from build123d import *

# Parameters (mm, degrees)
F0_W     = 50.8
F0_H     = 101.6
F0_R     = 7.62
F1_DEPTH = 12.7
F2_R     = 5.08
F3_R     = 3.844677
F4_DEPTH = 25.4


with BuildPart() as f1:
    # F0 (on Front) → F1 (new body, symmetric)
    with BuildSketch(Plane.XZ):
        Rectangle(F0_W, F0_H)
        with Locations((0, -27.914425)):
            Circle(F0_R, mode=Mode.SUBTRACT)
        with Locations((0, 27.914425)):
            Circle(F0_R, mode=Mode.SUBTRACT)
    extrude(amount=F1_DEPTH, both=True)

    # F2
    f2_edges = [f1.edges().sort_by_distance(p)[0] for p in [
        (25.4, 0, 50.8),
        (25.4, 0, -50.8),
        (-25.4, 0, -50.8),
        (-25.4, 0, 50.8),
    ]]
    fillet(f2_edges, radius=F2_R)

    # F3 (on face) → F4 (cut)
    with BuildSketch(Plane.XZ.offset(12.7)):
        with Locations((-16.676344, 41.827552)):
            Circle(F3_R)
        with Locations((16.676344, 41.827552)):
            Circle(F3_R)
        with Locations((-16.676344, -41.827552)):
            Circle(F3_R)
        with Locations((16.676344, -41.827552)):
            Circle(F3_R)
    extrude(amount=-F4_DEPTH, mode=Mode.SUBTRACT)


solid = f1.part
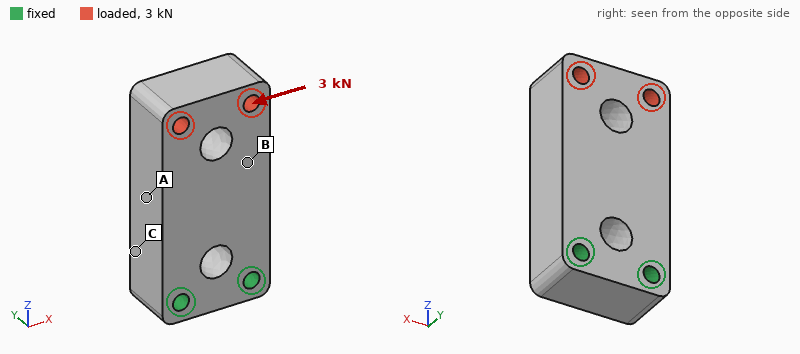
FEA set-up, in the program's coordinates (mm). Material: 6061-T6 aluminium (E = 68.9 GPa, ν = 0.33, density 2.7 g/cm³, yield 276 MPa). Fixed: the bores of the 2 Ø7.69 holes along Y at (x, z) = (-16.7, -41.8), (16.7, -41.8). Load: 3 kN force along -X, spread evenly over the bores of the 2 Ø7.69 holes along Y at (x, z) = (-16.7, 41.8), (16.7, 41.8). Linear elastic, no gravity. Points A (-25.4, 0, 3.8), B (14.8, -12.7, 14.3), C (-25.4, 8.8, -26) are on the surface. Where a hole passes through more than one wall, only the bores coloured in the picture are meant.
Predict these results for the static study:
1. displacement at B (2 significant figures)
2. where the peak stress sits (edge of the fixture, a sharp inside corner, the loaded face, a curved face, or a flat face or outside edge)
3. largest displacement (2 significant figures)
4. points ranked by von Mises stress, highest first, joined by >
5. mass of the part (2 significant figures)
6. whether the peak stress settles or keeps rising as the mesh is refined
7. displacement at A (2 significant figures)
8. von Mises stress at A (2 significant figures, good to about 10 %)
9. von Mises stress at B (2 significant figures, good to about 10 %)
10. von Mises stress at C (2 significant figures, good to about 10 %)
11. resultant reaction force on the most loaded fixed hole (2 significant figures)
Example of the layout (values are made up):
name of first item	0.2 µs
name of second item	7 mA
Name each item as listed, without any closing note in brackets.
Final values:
displacement at B	25 µm
where the peak stress sits	edge of the fixture
largest displacement	51 µm
points ranked by von Mises stress, highest first, joined by >	C > A > B
mass of the part	310 g
whether the peak stress settles or keeps rising as the mesh is refined	keeps rising
displacement at A	22 µm
von Mises stress at A	11 MPa
von Mises stress at B	4.9 MPa
von Mises stress at C	17 MPa
resultant reaction force on the most loaded fixed hole	6.6 kN
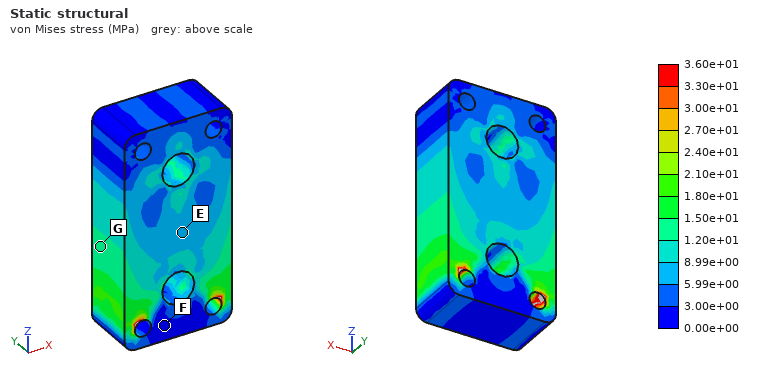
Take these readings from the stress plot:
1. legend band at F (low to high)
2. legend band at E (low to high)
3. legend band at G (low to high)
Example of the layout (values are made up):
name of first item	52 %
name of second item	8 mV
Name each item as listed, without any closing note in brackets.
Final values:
legend band at F	0.00e+00 to 3.00e+00 MPa
legend band at E	5.99e+00 to 8.99e+00 MPa
legend band at G	1.20e+01 to 1.50e+01 MPa
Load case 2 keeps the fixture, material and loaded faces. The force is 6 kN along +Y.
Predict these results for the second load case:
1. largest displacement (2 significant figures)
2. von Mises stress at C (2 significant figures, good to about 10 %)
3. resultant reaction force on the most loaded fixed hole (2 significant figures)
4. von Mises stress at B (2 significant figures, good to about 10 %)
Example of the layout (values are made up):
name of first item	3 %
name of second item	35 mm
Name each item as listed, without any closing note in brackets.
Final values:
largest displacement	0.37 mm
von Mises stress at C	59 MPa
resultant reaction force on the most loaded fixed hole	3.0 kN
von Mises stress at B	35 MPa
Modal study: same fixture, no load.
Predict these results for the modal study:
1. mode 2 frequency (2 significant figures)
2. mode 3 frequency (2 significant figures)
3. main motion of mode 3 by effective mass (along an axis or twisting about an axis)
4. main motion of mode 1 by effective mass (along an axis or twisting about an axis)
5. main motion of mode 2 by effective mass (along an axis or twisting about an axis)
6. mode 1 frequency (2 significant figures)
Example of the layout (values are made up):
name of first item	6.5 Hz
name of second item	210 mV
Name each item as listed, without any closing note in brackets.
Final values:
mode 2 frequency	4100 Hz
mode 3 frequency	6500 Hz
main motion of mode 3 by effective mass	twisting about Z
main motion of mode 1 by effective mass	along Y
main motion of mode 2 by effective mass	along X
mode 1 frequency	2200 Hz
